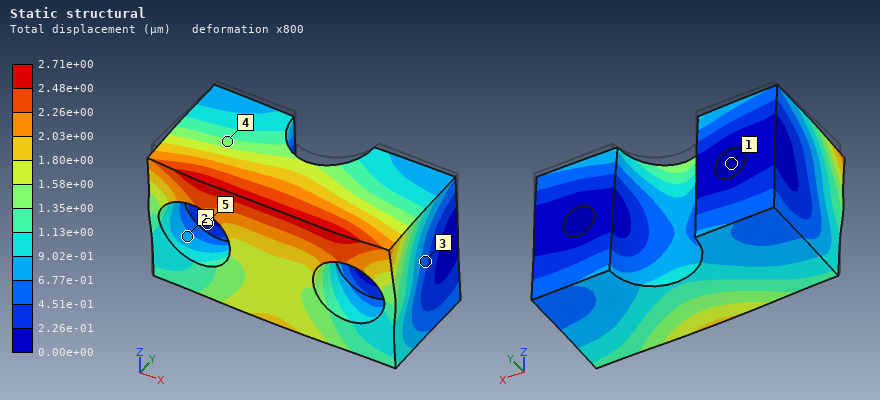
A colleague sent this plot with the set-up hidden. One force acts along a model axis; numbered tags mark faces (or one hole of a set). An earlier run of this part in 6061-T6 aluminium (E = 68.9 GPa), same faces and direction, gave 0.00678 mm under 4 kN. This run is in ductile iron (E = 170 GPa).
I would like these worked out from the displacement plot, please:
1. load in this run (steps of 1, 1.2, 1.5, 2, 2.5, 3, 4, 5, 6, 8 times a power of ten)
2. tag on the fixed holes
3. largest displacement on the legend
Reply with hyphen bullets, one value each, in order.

- 4 kN
- 1
- 2.71e+00 µm
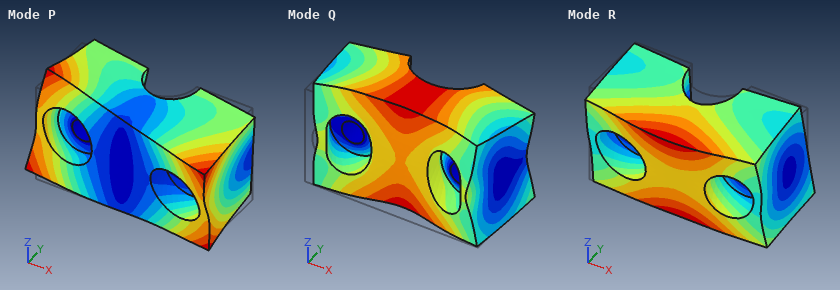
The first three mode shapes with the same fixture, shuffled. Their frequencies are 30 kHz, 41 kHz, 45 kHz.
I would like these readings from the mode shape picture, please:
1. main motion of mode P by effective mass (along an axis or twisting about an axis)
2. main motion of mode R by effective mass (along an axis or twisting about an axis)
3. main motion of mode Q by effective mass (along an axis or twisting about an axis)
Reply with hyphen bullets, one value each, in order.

- twisting about Y
- along Z
- along Y
